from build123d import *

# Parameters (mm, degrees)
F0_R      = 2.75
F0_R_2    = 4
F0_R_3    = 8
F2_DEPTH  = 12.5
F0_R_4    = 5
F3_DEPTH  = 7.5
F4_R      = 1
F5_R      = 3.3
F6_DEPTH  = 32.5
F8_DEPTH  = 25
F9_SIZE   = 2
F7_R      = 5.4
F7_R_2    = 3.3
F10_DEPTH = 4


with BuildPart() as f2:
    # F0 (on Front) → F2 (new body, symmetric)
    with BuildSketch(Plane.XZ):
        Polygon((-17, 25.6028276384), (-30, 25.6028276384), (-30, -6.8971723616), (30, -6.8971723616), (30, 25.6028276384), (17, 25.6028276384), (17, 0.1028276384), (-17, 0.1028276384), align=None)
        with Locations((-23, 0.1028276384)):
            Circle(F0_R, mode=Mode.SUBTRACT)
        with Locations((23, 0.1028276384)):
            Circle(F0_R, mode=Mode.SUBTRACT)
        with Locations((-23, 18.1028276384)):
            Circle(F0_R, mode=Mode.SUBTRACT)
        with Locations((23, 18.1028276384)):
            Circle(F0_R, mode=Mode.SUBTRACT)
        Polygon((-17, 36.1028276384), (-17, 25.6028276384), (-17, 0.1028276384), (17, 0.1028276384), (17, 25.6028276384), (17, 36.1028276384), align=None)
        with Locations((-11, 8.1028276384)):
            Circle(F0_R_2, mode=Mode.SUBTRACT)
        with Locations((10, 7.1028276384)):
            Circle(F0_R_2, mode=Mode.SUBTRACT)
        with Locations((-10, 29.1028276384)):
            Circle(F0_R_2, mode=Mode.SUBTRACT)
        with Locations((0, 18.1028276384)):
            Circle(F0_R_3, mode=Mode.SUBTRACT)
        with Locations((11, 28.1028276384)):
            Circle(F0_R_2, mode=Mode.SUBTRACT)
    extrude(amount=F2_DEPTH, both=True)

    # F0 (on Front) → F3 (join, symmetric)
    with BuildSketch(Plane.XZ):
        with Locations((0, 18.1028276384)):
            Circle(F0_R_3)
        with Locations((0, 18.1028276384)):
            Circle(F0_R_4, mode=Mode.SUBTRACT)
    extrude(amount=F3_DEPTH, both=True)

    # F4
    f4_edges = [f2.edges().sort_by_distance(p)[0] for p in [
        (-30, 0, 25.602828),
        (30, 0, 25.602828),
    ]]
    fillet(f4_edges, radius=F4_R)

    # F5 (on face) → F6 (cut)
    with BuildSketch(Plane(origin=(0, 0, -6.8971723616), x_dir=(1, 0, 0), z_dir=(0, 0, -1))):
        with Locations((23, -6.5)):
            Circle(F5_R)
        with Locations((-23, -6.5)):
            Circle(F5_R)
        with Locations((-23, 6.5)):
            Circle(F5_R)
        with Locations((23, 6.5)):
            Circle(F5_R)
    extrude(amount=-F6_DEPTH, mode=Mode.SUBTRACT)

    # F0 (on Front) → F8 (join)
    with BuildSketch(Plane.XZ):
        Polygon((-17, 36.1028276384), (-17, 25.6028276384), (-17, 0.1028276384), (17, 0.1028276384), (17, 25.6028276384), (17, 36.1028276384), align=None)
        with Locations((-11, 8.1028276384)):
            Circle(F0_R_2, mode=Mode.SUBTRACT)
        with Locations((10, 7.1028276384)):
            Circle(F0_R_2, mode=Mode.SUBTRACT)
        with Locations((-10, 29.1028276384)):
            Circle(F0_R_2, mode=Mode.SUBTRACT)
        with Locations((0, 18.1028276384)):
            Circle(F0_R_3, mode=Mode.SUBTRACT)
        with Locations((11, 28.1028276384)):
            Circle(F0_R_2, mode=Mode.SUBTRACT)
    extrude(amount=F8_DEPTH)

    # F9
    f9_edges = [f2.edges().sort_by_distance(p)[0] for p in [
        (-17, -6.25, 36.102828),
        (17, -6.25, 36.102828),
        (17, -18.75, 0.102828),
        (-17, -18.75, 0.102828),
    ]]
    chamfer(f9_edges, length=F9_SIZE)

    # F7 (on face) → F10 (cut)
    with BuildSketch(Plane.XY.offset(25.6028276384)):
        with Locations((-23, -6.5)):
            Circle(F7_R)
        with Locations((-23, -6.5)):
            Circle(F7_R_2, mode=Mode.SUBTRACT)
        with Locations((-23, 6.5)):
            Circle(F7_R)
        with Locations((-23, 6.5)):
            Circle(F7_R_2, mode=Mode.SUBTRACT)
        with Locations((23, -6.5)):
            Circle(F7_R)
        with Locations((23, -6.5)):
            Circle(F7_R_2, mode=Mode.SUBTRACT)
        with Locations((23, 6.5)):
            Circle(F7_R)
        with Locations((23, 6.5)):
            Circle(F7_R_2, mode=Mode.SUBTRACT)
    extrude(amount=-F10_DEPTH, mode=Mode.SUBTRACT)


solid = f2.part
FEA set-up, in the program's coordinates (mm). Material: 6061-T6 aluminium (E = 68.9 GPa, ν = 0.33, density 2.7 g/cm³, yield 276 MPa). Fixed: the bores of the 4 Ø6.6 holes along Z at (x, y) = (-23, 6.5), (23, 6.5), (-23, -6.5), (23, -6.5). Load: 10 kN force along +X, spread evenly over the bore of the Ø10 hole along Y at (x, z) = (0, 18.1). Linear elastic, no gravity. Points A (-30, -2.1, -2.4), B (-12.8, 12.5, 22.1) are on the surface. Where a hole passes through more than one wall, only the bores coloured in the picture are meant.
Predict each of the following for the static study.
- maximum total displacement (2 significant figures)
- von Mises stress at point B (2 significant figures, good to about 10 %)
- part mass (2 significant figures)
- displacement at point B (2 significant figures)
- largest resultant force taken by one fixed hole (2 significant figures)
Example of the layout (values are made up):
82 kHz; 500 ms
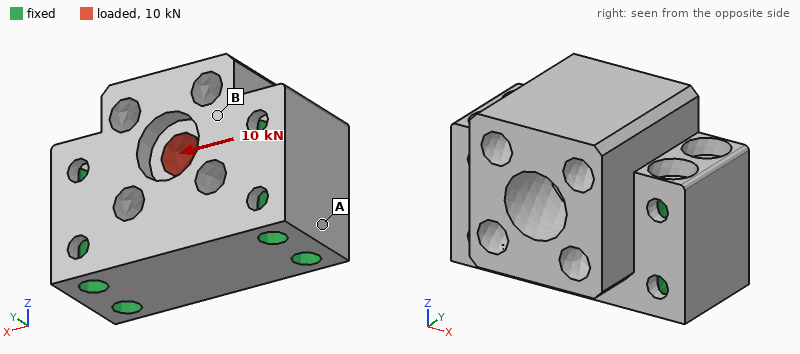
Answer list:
6.1 µm; 12 MPa; 140 g; 2.4 µm; 2.7 kN
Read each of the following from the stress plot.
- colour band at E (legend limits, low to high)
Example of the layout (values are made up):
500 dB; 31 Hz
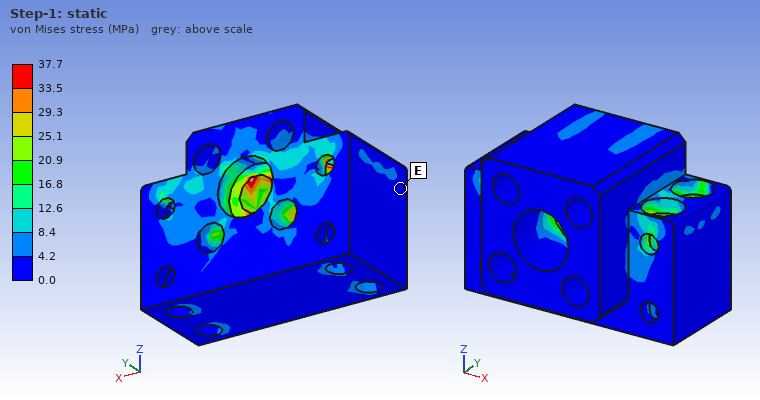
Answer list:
0.0 to 4.2 MPa
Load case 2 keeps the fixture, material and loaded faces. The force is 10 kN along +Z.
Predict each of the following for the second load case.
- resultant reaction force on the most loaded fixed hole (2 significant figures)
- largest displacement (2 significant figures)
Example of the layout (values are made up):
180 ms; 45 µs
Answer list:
2.6 kN; 9.6 µm
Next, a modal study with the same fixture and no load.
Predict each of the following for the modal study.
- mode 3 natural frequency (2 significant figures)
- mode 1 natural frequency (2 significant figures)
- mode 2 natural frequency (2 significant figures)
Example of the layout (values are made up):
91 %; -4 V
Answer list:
24 kHz; 14 kHz; 24 kHz
